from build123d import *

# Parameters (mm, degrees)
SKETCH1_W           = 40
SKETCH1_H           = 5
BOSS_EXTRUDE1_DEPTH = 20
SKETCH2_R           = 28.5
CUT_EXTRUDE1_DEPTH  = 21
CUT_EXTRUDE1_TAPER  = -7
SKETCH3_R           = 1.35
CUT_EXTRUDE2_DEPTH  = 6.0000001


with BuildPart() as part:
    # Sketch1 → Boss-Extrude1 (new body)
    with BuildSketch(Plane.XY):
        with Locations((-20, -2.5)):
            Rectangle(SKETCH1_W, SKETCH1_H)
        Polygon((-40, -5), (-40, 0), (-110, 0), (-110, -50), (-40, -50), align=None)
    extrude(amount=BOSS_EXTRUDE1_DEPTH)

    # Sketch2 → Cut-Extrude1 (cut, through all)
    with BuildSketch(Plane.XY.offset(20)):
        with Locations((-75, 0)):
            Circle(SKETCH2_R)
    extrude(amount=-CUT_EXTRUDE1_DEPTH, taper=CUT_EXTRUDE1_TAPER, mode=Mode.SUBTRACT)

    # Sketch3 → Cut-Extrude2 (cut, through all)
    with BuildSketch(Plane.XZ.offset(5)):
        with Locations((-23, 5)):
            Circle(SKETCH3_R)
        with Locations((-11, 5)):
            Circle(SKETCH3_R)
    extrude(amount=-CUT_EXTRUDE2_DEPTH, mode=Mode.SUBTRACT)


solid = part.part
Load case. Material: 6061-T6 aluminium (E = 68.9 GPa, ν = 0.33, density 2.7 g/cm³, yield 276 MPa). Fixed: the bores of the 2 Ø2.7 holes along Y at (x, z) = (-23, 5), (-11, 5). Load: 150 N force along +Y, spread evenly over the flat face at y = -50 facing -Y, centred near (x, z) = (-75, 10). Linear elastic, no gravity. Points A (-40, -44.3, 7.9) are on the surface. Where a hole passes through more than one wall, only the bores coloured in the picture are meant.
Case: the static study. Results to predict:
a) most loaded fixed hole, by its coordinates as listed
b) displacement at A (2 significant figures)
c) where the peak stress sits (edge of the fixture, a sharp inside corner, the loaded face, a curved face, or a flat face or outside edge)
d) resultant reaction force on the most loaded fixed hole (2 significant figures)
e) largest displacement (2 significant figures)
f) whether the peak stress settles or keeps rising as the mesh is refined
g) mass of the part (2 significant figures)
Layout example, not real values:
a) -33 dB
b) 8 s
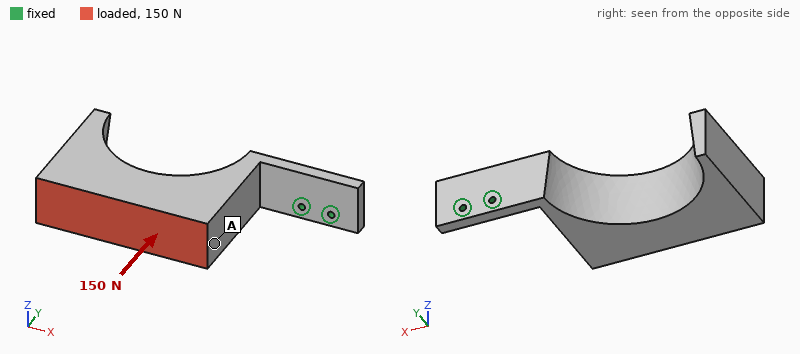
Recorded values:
a) (-23, 5)
b) 0.46 mm
c) edge of the fixture
d) 420 N
e) 1.0 mm
f) keeps rising
g) 120 g
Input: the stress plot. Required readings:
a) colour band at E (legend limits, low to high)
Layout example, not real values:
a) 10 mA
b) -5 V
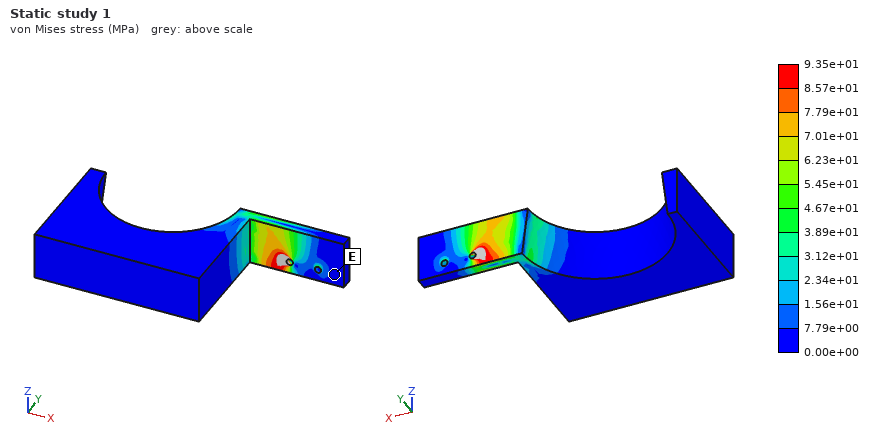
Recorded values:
a) 0.00e+00 to 7.79e+00 MPa
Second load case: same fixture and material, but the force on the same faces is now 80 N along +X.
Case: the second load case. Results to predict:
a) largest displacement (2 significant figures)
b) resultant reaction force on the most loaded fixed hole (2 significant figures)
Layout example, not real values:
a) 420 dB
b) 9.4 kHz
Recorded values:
a) 0.60 mm
b) 150 N
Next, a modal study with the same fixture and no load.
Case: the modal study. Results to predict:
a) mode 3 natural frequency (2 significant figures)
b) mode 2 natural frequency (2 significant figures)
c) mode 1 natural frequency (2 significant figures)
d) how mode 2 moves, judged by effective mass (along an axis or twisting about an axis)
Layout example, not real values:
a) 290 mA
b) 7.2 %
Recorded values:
a) 920 Hz
b) 380 Hz
c) 190 Hz
d) along Z
